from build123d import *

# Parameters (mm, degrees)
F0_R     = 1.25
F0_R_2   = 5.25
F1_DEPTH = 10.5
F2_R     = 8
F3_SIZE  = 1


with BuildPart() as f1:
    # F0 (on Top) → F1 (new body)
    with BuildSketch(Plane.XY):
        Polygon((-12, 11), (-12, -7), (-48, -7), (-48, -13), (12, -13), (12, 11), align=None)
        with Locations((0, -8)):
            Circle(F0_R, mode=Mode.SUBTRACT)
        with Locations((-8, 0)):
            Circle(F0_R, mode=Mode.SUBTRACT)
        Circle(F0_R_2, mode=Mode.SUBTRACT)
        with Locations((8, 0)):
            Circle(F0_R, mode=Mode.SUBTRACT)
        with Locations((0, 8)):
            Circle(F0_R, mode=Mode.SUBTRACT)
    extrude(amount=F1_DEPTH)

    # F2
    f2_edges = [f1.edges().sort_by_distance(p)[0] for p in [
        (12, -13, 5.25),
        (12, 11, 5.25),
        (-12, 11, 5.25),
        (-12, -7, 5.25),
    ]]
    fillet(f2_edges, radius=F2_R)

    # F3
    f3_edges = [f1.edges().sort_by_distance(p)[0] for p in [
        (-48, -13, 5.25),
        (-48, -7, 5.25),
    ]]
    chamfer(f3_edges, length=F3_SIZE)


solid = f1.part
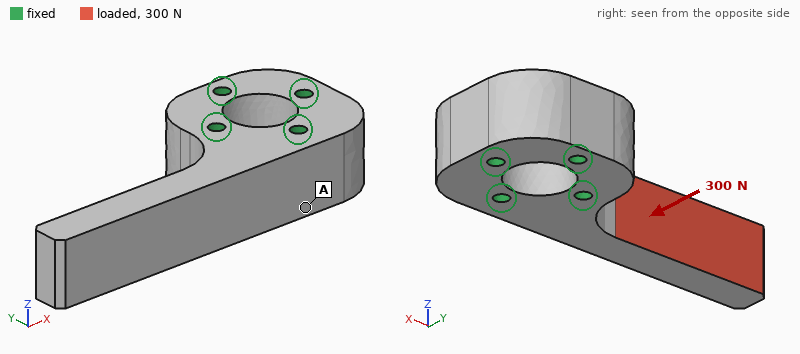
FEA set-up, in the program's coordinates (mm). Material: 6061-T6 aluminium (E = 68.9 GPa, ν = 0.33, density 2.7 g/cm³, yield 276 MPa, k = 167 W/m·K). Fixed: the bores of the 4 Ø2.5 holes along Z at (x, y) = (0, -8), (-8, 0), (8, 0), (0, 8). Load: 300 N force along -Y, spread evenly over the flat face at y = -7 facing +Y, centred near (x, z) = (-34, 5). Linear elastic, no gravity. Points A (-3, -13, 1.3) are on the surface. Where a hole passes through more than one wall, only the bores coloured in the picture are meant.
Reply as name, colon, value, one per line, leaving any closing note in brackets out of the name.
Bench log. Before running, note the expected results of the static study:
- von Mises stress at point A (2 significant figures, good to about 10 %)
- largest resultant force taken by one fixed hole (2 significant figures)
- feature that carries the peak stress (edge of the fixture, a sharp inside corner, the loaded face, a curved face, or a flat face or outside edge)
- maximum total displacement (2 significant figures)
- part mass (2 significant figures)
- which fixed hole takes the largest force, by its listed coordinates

von Mises stress at point A: 10 MPa
largest resultant force taken by one fixed hole: 770 N
feature that carries the peak stress: a curved face
maximum total displacement: 0.15 mm
part mass: 19 g
which fixed hole takes the largest force, by its listed coordinates: (-8, 0)
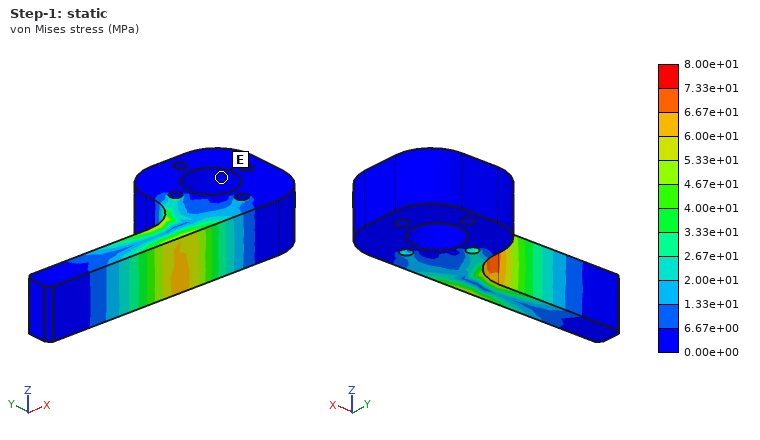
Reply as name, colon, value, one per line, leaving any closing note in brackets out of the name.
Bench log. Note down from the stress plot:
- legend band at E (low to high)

legend band at E: 0.00e+00 to 6.67e+00 MPa
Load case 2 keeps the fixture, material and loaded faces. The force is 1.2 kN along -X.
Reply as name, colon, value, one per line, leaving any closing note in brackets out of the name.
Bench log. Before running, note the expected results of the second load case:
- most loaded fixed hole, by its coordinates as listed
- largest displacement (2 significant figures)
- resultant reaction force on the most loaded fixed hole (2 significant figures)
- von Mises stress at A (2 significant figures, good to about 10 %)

most loaded fixed hole, by its coordinates as listed: (0, -8)
largest displacement: 0.11 mm
resultant reaction force on the most loaded fixed hole: 830 N
von Mises stress at A: 7.4 MPa
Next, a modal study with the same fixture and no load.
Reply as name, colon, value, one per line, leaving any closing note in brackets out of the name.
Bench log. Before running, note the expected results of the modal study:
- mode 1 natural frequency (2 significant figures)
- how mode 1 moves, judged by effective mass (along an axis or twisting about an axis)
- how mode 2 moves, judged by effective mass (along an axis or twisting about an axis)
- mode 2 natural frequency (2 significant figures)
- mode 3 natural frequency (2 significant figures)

mode 1 natural frequency: 4000 Hz
how mode 1 moves, judged by effective mass: along Y
how mode 2 moves, judged by effective mass: along Z
mode 2 natural frequency: 5000 Hz
mode 3 natural frequency: 18 kHz
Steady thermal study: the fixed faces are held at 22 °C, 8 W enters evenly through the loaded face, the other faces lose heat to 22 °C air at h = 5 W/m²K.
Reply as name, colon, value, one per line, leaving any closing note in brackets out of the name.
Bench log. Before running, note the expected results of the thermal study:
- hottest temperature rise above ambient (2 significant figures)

hottest temperature rise above ambient: 19 K
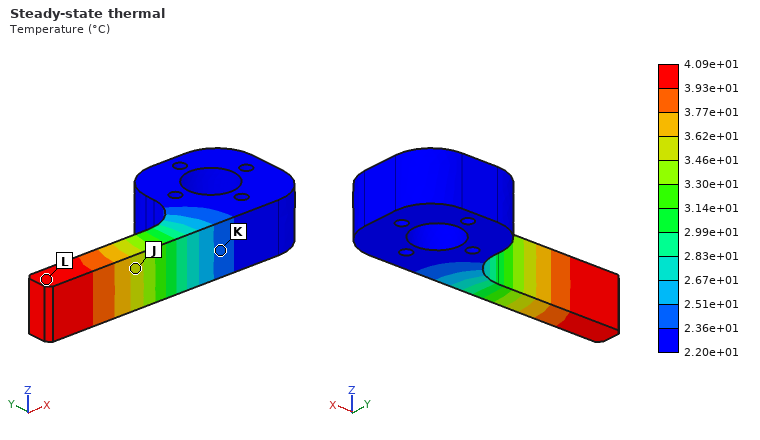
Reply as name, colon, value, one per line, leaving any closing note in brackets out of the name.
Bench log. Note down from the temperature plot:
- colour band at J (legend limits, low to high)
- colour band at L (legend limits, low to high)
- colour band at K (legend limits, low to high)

colour band at J: 3.46e+01 to 3.62e+01 °C
colour band at L: 3.93e+01 to 4.09e+01 °C
colour band at K: 2.36e+01 to 2.51e+01 °C
